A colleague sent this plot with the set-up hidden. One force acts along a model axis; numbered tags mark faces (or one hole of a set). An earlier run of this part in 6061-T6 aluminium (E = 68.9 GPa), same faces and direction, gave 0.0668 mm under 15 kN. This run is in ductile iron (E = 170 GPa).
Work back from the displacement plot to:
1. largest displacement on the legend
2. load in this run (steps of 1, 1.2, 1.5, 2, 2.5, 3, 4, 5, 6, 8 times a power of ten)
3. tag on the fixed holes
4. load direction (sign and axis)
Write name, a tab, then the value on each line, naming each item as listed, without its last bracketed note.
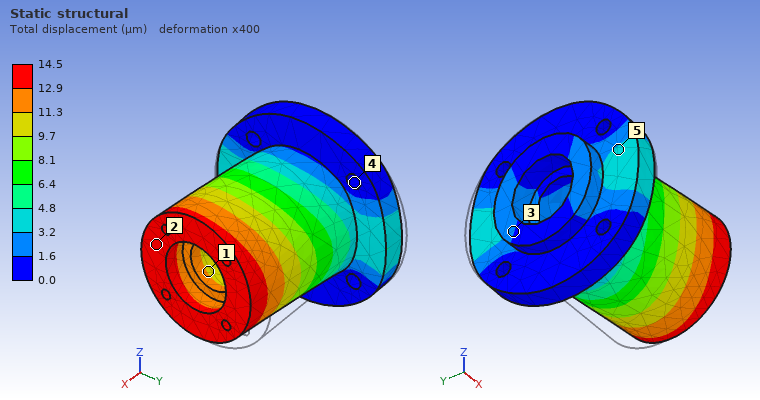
largest displacement on the legend	14.5 µm
load in this run	8 kN
tag on the fixed holes	4
load direction	-Y
